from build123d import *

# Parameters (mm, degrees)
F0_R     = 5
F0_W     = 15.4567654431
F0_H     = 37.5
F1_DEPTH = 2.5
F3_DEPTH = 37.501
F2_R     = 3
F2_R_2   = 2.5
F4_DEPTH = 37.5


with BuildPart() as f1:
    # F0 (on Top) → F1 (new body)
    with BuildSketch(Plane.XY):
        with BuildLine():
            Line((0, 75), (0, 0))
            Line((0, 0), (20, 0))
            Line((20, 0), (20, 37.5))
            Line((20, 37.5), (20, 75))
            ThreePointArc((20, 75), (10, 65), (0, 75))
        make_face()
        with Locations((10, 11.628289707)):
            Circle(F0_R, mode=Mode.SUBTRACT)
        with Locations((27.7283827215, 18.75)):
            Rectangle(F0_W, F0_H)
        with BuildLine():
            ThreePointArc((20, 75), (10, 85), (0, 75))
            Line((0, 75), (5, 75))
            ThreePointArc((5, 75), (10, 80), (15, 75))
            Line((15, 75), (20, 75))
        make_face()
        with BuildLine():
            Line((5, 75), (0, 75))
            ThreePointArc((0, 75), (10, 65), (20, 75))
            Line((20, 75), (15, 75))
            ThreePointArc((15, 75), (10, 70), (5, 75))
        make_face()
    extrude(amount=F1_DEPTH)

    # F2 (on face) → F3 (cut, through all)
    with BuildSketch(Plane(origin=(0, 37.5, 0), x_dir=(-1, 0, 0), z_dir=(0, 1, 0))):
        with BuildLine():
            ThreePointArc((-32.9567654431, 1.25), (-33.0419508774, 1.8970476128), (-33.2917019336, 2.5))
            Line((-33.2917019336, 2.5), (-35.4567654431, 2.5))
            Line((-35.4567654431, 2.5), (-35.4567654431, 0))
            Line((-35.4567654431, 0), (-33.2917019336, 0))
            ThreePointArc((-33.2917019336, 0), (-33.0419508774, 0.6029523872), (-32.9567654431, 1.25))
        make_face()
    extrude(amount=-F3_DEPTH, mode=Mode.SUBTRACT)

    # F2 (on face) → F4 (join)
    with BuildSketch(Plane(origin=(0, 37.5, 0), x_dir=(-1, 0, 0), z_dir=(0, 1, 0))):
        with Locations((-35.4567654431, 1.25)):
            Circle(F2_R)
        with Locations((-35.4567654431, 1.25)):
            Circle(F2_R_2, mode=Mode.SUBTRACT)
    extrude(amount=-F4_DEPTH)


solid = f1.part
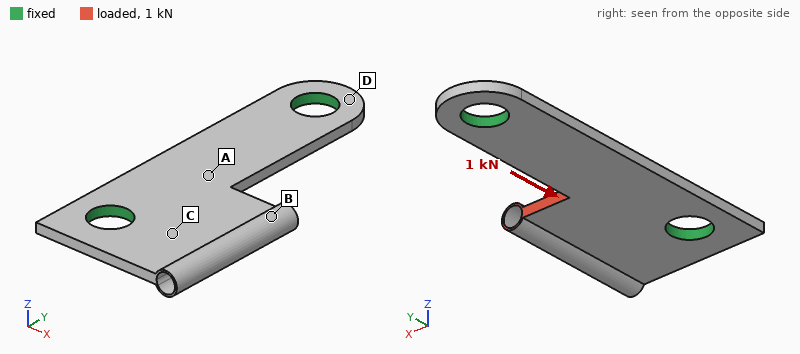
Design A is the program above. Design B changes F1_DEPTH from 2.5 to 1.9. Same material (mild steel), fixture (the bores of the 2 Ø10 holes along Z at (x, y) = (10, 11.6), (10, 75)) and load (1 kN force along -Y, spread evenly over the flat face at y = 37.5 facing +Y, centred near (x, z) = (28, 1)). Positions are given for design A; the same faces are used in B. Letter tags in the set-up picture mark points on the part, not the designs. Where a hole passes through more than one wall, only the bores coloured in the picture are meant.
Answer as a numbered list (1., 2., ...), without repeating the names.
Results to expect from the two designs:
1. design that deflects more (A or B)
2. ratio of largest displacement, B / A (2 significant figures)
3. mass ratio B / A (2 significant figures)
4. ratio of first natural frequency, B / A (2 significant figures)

1. B
2. 1.4
3. 0.77
4. 0.73
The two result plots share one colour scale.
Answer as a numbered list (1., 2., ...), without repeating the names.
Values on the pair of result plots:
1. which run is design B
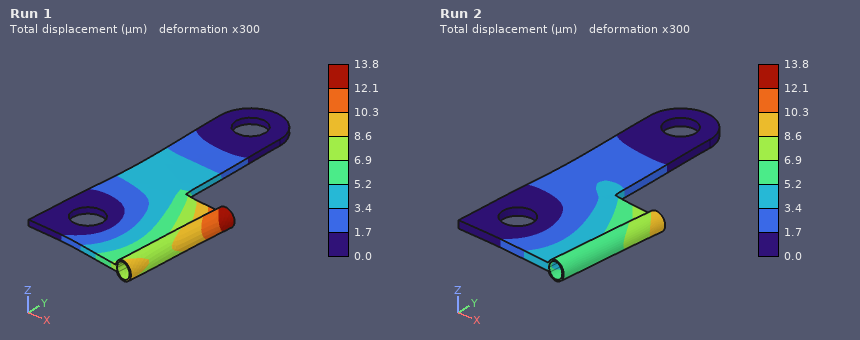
1. Run 1
